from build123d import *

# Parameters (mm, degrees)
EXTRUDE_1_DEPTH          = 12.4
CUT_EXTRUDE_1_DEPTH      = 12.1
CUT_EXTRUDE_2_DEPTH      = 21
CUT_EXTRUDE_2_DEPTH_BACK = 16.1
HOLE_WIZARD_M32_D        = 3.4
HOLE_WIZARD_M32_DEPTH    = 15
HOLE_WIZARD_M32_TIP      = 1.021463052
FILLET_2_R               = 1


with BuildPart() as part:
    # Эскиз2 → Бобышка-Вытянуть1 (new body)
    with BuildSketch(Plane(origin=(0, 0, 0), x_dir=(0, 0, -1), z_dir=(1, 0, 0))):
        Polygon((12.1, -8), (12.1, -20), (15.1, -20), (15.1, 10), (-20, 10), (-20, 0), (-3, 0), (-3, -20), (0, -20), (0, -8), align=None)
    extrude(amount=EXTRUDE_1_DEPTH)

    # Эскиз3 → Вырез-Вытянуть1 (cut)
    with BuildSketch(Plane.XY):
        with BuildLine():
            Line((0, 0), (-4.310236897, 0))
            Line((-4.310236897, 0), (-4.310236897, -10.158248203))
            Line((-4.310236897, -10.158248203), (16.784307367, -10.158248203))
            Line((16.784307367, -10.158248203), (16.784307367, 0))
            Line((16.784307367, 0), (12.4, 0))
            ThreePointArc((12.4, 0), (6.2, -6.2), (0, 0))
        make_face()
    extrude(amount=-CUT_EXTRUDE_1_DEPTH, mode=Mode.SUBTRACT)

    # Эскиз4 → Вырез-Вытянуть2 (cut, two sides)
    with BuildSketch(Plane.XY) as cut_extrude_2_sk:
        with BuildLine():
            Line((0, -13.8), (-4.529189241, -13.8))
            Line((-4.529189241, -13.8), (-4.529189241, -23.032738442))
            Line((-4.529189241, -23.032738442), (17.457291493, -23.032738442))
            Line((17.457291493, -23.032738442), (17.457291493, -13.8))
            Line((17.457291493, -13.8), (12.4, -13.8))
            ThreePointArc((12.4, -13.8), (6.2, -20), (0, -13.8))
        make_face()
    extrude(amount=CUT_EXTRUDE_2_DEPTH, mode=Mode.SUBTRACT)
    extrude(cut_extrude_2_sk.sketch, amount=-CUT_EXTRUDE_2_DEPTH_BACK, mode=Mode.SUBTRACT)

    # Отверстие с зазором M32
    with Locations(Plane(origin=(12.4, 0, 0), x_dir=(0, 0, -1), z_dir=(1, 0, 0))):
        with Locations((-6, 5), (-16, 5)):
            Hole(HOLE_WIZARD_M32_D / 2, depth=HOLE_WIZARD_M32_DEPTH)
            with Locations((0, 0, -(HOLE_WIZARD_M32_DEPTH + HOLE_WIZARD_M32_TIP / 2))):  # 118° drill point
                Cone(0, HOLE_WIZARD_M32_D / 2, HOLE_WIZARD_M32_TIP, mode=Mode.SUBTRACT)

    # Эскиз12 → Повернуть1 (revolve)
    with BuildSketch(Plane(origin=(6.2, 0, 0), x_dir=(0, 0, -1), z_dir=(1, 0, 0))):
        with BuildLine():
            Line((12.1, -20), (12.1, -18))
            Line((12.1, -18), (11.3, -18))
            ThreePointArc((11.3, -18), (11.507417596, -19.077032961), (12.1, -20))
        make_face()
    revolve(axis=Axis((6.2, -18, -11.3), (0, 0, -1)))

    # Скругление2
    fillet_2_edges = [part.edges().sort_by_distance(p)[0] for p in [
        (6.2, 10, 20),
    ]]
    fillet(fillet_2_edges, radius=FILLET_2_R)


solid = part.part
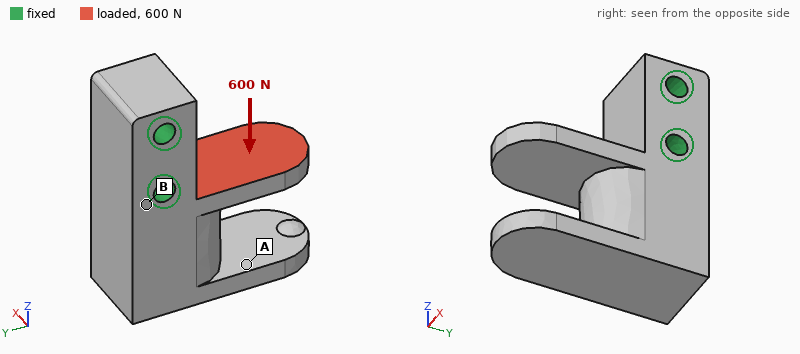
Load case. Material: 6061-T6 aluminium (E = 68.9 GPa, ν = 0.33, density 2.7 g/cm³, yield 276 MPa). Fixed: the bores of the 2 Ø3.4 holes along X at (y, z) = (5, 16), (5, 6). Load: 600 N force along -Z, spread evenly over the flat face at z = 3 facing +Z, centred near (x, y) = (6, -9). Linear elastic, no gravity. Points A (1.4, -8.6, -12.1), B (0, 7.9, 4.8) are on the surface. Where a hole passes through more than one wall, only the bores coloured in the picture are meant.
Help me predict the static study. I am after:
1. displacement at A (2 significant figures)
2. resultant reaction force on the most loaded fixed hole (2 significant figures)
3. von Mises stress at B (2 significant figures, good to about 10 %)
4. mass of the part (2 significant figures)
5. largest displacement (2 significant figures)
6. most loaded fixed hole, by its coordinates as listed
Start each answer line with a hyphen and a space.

- 0.025 mm
- 650 N
- 21 MPa
- 17 g
- 0.15 mm
- (5, 6)
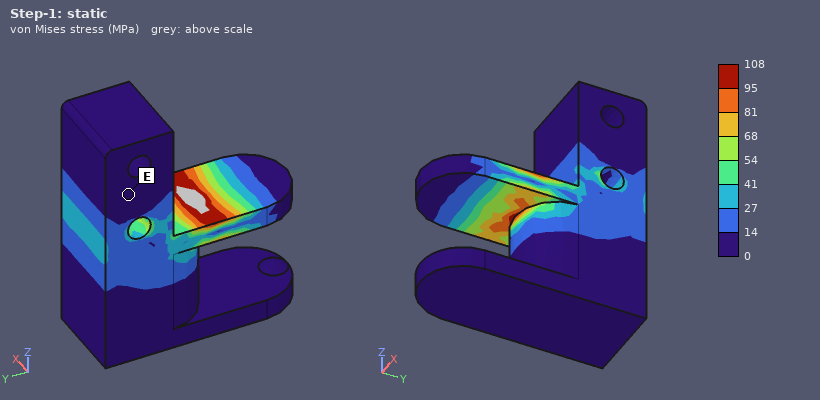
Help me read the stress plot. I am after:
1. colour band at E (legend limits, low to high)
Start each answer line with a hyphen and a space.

- 0 to 14 MPa
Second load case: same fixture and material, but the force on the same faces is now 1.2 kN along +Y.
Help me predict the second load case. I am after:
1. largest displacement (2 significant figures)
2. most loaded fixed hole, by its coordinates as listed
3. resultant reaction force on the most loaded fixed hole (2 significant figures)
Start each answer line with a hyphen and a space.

- 68 µm
- (5, 6)
- 1.3 kN
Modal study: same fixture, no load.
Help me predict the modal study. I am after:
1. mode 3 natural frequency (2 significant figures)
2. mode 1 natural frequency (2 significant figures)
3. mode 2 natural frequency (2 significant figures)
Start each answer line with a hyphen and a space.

- 11 kHz
- 7300 Hz
- 11 kHz
